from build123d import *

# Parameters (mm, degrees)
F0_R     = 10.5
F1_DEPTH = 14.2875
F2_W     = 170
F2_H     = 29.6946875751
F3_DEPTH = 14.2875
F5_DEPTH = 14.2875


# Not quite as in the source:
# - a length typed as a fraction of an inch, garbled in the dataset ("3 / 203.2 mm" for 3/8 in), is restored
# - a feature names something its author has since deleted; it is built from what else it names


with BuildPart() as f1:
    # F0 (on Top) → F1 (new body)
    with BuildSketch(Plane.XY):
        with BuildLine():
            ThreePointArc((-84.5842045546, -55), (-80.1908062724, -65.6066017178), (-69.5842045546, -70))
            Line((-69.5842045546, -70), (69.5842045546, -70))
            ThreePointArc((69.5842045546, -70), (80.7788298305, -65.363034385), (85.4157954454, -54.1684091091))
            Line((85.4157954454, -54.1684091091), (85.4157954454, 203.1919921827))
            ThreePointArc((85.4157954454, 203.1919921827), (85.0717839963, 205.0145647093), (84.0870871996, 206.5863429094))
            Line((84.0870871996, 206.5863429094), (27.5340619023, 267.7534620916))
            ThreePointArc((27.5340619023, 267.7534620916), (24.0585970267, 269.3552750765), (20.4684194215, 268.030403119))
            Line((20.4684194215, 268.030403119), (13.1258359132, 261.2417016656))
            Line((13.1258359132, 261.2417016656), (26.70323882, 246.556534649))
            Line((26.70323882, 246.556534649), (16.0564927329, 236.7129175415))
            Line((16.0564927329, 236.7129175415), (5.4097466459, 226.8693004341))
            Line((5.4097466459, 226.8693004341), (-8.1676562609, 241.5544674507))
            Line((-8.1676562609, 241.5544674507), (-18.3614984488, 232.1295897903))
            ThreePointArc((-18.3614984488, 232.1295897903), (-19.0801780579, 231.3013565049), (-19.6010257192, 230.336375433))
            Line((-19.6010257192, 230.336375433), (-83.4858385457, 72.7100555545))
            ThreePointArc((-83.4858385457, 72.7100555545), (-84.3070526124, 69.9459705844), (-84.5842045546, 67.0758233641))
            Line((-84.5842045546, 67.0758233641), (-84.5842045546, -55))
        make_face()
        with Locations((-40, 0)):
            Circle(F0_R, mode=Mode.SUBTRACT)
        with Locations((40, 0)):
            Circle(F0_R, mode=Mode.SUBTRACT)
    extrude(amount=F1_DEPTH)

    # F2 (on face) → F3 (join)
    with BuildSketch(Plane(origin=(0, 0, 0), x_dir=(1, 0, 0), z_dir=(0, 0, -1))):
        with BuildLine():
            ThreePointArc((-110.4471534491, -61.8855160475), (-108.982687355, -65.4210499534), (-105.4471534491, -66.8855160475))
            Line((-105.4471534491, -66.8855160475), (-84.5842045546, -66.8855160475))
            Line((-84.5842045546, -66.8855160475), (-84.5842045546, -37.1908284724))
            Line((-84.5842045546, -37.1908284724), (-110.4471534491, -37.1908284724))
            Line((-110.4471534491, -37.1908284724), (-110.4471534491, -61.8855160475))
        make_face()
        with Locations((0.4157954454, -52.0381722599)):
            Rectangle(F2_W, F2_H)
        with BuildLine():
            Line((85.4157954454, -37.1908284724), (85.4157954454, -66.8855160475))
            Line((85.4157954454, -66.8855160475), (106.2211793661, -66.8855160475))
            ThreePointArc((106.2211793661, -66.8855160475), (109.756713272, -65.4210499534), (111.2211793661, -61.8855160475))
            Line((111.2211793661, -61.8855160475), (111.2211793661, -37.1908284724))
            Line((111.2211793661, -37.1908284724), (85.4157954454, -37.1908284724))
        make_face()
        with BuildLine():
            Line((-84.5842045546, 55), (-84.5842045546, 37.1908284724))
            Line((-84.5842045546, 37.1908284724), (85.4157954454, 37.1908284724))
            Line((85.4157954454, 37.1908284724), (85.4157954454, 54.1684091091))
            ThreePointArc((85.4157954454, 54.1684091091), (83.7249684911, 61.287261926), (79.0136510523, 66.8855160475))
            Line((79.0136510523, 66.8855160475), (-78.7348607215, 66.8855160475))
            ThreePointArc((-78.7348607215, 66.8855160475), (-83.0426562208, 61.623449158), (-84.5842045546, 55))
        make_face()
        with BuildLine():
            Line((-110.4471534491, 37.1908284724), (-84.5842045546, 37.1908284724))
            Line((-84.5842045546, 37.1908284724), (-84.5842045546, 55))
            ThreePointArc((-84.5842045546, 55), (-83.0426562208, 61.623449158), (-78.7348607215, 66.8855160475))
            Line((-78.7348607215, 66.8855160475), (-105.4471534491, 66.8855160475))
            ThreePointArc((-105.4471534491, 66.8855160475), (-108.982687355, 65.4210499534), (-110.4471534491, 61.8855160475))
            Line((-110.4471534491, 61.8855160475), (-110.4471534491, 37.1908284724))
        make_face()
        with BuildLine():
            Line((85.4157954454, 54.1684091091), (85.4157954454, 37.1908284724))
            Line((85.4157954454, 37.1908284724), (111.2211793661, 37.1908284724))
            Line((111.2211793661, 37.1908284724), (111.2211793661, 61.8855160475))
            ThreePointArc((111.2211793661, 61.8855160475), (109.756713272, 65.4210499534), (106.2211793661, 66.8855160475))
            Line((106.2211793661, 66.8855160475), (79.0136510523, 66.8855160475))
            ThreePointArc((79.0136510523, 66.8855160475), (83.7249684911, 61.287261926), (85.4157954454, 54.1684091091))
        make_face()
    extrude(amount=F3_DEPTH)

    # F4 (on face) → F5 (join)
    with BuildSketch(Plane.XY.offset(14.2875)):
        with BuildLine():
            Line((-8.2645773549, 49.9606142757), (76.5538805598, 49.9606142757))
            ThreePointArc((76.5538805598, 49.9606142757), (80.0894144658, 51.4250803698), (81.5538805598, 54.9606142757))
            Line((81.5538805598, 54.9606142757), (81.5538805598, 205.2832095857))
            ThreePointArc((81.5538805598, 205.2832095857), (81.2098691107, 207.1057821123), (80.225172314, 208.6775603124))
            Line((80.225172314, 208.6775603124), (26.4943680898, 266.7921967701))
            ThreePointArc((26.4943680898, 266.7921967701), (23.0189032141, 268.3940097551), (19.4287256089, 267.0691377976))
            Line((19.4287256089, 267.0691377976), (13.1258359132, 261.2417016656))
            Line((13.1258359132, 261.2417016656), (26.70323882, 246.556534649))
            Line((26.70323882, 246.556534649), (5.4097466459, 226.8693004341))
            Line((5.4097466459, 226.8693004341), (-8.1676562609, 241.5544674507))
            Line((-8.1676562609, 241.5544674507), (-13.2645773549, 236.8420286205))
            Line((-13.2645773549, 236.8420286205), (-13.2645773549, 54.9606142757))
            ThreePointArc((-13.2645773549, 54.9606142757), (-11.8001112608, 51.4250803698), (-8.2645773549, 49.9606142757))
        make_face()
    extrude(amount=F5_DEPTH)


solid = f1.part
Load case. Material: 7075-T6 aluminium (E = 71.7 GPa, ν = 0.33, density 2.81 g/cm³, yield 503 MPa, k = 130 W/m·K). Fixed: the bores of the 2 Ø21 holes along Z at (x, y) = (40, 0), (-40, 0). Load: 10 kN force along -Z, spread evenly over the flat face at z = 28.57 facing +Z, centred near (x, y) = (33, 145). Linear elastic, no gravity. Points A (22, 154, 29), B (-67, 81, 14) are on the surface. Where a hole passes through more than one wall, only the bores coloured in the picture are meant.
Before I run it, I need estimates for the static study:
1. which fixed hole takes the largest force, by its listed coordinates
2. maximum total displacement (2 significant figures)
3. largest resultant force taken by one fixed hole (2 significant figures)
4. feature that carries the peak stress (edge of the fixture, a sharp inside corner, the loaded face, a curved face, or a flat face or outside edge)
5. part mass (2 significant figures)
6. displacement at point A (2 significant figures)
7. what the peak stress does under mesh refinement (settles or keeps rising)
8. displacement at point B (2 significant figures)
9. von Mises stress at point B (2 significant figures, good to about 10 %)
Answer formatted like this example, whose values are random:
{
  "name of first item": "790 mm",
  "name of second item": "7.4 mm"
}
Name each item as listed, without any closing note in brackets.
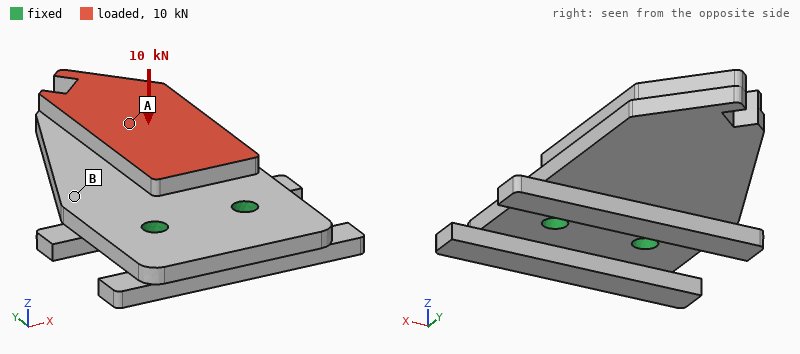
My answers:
{
  "which fixed hole takes the largest force, by its listed coordinates": "(40, 0)",
  "maximum total displacement": "4.9 mm",
  "largest resultant force taken by one fixed hole": "8.2 kN",
  "feature that carries the peak stress": "edge of the fixture",
  "part mass": "3.1 kg",
  "displacement at point A": "2.5 mm",
  "what the peak stress does under mesh refinement": "keeps rising",
  "displacement at point B": "0.82 mm",
  "von Mises stress at point B": "57 MPa"
}
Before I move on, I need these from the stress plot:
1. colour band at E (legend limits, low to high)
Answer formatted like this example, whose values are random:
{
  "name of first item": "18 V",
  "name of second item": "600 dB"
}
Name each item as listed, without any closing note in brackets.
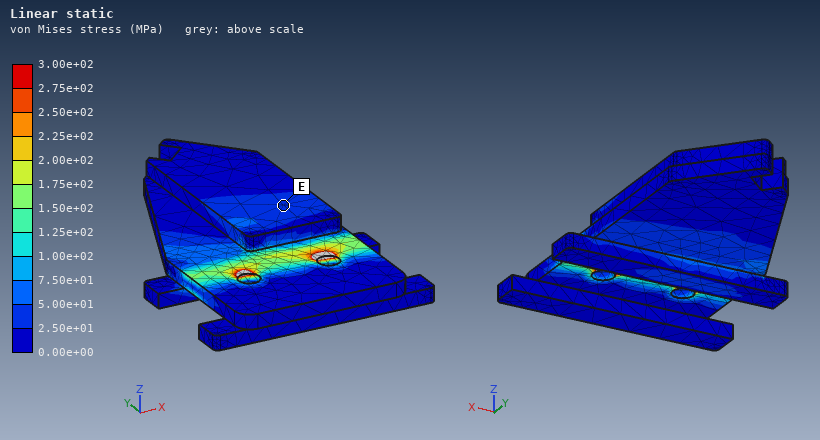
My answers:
{
  "colour band at E": "2.50e+01 to 5.00e+01 MPa"
}
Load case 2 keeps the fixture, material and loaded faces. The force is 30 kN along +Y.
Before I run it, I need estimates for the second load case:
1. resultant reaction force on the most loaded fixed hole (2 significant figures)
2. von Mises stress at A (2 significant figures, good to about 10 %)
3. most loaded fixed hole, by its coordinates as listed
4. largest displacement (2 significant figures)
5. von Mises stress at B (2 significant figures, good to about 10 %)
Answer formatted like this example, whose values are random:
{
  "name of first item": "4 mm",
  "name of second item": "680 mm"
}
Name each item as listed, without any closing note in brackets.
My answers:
{
  "resultant reaction force on the most loaded fixed hole": "26 kN",
  "von Mises stress at A": "21 MPa",
  "most loaded fixed hole, by its coordinates as listed": "(40, 0)",
  "largest displacement": "2.7 mm",
  "von Mises stress at B": "34 MPa"
}
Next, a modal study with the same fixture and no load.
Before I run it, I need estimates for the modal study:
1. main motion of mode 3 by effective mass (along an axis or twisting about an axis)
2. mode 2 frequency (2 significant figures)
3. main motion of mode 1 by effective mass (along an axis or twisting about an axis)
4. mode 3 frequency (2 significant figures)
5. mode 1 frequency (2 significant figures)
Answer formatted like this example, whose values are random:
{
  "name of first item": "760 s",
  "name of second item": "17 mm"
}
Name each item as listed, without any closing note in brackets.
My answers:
{
  "main motion of mode 3 by effective mass": "along X",
  "mode 2 frequency": "1300 Hz",
  "main motion of mode 1 by effective mass": "along Z",
  "mode 3 frequency": "1500 Hz",
  "mode 1 frequency": "230 Hz"
}
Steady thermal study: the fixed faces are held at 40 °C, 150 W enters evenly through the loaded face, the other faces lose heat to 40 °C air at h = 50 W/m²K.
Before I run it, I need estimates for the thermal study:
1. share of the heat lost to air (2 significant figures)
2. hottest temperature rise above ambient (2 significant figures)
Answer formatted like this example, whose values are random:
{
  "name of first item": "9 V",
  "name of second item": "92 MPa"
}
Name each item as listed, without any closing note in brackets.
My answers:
{
  "share of the heat lost to air": "49 %",
  "hottest temperature rise above ambient": "33 K"
}
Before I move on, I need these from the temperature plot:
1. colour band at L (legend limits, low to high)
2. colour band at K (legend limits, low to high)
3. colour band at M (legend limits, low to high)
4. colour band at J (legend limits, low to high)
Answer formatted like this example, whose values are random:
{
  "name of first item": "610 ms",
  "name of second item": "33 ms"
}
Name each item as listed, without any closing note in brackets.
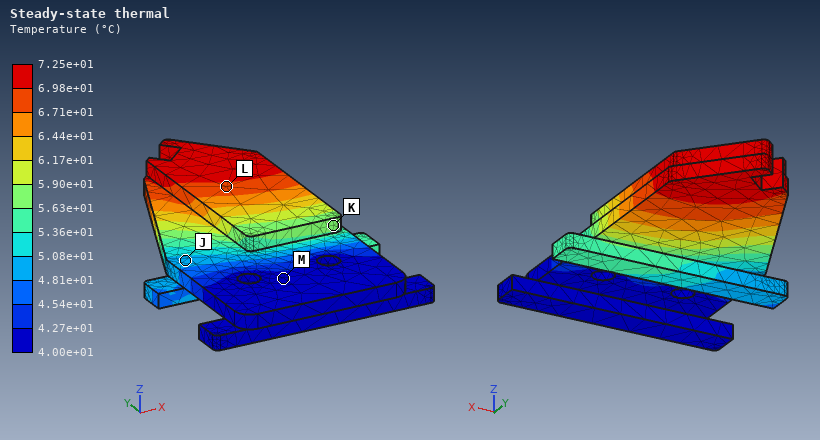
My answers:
{
  "colour band at L": "6.71e+01 to 6.98e+01 °C",
  "colour band at K": "5.63e+01 to 5.90e+01 °C",
  "colour band at M": "4.00e+01 to 4.27e+01 °C",
  "colour band at J": "4.81e+01 to 5.08e+01 °C"
}
